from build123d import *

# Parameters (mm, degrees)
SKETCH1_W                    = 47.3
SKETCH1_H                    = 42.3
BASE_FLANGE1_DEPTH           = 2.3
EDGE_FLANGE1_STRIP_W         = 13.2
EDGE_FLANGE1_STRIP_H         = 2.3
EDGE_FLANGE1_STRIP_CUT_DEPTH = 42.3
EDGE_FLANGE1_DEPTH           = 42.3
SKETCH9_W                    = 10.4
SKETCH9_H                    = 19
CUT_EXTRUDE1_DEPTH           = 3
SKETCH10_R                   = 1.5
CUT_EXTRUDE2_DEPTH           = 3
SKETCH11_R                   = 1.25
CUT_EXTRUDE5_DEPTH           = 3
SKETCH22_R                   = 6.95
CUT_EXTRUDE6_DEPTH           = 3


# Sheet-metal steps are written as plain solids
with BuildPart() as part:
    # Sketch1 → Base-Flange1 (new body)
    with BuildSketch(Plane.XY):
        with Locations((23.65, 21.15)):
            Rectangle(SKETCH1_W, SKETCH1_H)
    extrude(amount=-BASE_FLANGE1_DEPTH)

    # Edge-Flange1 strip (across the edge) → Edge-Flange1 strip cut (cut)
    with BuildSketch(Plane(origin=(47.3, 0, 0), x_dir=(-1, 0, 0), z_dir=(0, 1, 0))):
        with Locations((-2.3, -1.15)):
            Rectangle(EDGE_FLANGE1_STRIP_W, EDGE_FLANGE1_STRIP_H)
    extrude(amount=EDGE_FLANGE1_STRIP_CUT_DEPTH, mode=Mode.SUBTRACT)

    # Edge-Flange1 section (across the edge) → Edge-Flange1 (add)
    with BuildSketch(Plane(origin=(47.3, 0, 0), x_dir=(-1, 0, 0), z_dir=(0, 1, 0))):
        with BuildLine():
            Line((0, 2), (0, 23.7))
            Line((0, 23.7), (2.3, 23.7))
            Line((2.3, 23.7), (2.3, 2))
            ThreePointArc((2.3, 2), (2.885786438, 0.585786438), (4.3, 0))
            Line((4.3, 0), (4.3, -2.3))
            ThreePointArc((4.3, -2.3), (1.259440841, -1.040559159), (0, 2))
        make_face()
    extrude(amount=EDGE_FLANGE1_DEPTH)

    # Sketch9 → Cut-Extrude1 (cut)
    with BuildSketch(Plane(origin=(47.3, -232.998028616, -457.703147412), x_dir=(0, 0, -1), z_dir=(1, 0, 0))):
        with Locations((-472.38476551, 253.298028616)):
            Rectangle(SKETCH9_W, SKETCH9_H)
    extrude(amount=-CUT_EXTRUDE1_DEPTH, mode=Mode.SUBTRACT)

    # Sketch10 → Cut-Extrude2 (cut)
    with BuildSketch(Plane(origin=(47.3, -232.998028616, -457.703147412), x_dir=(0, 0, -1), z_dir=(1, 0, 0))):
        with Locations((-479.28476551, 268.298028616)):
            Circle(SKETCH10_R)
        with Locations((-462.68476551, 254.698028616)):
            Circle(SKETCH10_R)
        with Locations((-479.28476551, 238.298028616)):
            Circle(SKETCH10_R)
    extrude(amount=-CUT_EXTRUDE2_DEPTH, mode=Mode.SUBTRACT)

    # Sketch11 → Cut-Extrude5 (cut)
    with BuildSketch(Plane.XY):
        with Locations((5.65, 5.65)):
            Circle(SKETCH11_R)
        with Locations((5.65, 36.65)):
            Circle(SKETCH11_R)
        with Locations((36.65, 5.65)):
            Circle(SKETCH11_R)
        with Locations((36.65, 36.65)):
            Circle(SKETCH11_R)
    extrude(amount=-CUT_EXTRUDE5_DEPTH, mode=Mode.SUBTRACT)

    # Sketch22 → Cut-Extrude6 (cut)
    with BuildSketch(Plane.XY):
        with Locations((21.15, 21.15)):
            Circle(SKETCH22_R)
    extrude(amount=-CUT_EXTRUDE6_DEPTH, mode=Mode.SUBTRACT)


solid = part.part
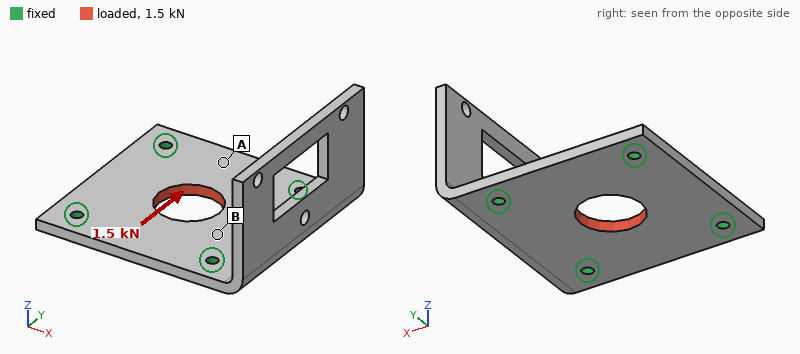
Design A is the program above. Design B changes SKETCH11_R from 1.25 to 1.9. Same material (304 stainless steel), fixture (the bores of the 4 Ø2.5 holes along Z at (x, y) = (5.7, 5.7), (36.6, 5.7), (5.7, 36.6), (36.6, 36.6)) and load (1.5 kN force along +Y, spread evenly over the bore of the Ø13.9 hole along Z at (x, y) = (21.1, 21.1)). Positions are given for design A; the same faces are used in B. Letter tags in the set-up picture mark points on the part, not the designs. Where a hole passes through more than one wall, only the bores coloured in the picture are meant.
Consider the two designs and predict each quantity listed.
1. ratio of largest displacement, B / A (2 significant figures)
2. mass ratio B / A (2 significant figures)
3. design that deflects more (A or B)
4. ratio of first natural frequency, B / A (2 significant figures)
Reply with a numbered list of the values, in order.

1. 0.92
2. 0.99
3. A
4. 1.0
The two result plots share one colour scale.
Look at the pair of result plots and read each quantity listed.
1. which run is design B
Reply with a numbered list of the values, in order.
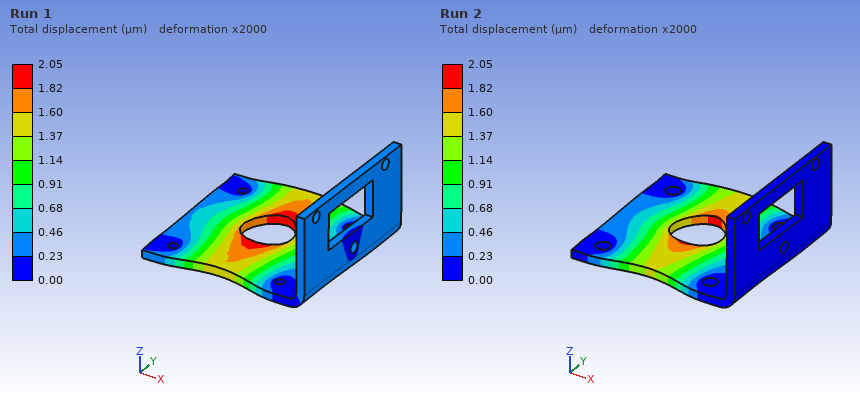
1. Run 2
